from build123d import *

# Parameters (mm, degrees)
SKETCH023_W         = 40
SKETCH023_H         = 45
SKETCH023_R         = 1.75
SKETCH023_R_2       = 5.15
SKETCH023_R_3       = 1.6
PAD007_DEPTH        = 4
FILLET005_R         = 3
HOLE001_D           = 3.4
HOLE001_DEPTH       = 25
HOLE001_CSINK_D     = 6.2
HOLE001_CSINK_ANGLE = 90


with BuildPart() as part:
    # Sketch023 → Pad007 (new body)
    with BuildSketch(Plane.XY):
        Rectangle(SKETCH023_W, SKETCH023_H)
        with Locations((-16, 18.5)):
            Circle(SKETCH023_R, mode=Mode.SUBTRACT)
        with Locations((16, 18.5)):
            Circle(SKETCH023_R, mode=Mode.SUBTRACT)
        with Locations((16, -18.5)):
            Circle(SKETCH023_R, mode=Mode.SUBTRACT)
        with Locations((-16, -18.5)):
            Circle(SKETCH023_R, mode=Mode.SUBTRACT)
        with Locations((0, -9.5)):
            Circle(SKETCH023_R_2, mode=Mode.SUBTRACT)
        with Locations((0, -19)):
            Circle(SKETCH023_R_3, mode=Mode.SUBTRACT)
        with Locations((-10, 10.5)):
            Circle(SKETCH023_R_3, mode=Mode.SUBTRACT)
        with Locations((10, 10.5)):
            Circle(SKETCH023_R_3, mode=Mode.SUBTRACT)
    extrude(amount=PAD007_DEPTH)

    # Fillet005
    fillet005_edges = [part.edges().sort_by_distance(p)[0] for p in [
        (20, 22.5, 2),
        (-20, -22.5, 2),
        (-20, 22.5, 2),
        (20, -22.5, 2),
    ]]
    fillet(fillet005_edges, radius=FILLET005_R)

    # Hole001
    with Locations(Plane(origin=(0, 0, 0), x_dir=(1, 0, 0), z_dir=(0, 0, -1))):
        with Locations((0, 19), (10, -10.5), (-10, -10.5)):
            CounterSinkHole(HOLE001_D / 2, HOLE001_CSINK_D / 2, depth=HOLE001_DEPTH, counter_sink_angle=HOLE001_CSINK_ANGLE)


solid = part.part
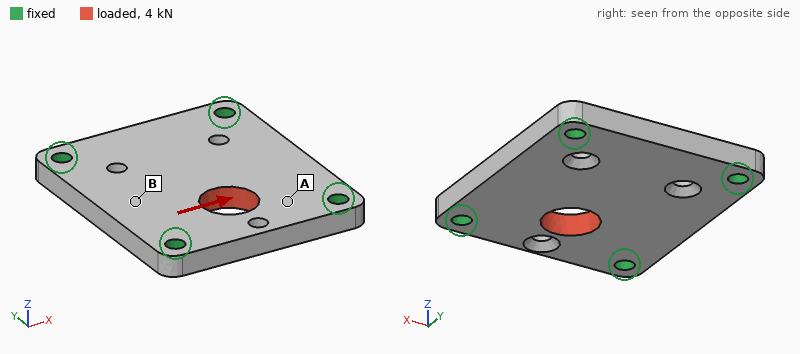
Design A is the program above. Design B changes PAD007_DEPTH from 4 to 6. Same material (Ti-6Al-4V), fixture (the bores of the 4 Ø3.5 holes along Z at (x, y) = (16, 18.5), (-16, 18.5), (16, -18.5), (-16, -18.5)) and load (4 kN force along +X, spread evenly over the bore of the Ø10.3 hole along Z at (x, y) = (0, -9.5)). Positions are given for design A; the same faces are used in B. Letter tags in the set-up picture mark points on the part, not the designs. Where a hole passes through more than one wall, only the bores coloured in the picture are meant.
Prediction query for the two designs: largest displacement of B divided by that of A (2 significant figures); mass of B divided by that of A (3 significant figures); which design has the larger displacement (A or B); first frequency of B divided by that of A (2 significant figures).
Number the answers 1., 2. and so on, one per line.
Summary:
1. 0.66
2. 1.50
3. A
4. 1.3
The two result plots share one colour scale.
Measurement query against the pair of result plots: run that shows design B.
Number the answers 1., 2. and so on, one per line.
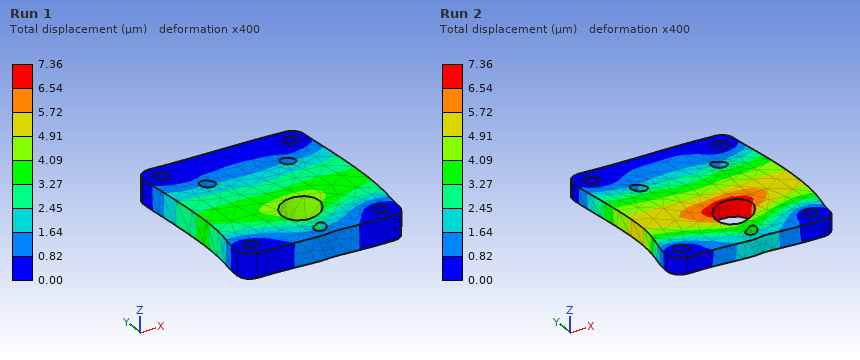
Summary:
1. Run 1
